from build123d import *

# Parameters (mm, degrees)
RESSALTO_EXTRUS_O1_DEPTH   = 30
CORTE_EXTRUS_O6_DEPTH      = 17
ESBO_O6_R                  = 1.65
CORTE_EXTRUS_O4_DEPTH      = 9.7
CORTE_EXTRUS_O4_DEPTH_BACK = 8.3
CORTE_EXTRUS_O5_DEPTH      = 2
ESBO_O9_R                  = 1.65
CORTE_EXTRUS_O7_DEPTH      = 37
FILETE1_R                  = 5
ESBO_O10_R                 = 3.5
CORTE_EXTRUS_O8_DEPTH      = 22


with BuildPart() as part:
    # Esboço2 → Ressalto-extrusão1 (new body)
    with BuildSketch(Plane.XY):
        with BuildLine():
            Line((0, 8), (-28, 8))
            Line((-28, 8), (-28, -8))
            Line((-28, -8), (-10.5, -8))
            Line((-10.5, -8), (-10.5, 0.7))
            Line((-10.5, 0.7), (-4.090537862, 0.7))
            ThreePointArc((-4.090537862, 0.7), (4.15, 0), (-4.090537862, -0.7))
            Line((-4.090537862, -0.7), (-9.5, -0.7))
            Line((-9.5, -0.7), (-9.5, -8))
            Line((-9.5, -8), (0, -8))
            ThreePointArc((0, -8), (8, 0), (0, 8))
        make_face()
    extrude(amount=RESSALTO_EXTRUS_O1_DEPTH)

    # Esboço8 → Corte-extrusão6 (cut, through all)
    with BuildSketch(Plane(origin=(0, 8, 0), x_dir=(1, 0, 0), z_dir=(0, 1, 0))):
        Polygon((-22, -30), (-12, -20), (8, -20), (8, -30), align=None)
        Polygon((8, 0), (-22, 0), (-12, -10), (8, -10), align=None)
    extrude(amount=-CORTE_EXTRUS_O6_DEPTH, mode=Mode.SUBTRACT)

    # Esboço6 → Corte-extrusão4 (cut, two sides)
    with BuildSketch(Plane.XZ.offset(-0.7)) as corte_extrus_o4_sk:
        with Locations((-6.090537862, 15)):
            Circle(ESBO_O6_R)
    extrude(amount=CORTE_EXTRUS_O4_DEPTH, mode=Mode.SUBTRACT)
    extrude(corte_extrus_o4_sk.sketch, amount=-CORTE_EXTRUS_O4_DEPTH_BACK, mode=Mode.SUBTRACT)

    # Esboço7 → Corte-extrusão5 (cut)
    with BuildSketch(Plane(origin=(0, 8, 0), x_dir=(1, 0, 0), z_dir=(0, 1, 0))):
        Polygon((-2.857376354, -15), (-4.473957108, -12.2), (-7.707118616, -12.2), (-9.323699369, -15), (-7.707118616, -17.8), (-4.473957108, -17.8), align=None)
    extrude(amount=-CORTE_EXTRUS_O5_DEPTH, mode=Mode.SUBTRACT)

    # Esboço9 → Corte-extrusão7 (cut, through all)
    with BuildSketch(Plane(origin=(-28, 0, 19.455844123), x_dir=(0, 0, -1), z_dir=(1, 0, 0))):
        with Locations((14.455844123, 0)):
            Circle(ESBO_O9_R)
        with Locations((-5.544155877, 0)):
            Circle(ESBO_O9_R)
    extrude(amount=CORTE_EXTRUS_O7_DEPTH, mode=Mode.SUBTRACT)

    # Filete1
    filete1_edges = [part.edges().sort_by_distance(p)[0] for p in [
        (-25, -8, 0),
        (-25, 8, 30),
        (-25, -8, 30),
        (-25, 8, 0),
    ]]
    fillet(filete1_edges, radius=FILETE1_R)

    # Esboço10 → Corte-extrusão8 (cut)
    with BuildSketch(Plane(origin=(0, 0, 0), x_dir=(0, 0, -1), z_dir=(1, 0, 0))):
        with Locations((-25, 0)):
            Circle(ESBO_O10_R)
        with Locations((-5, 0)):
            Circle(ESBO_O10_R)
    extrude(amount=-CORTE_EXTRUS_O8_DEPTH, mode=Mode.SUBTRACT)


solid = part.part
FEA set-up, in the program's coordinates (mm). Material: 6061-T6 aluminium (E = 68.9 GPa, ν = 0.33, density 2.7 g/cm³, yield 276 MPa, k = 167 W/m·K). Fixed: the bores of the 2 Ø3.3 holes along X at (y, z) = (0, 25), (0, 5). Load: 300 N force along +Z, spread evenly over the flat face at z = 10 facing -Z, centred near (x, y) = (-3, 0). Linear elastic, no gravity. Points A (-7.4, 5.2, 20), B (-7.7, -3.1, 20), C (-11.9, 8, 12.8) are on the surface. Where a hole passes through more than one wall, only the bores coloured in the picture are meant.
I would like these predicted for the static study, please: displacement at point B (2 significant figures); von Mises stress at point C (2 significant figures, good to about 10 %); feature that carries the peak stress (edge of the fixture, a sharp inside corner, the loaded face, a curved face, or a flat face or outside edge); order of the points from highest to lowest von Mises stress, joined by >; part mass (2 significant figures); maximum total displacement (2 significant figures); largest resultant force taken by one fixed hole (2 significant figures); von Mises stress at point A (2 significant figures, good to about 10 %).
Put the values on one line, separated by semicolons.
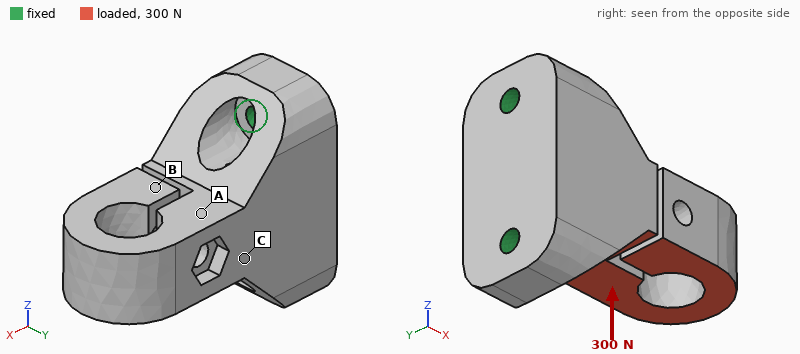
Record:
0.081 mm; 13 MPa; a curved face; A > C > B; 20 g; 0.10 mm; 350 N; 26 MPa
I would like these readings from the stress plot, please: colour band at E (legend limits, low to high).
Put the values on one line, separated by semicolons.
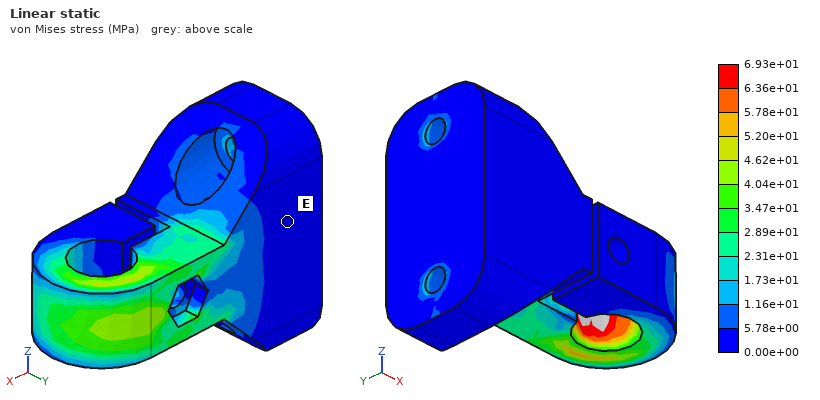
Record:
0.00e+00 to 5.78e+00 MPa
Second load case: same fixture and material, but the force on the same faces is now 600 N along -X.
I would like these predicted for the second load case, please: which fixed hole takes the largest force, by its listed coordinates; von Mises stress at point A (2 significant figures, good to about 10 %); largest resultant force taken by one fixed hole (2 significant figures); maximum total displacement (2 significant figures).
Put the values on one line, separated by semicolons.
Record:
(0, 5); 25 MPa; 460 N; 0.22 mm
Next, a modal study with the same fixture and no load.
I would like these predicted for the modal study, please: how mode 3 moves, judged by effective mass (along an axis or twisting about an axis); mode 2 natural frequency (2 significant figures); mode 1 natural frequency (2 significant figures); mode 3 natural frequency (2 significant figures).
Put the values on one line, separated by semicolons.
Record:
along Y; 4400 Hz; 4000 Hz; 5500 Hz
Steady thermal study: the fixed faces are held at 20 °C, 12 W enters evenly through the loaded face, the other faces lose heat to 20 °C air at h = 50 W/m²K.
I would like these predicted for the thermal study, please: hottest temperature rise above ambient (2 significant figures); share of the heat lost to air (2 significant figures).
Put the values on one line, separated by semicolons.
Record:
32 K; 13 %
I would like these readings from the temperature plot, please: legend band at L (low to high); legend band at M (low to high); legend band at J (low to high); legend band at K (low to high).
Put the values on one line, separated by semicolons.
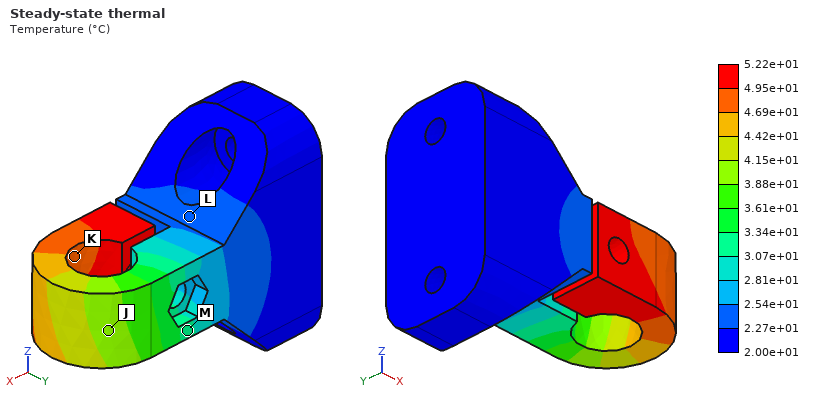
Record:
2.27e+01 to 2.54e+01 °C; 3.07e+01 to 3.34e+01 °C; 3.88e+01 to 4.15e+01 °C; 4.69e+01 to 4.95e+01 °C
